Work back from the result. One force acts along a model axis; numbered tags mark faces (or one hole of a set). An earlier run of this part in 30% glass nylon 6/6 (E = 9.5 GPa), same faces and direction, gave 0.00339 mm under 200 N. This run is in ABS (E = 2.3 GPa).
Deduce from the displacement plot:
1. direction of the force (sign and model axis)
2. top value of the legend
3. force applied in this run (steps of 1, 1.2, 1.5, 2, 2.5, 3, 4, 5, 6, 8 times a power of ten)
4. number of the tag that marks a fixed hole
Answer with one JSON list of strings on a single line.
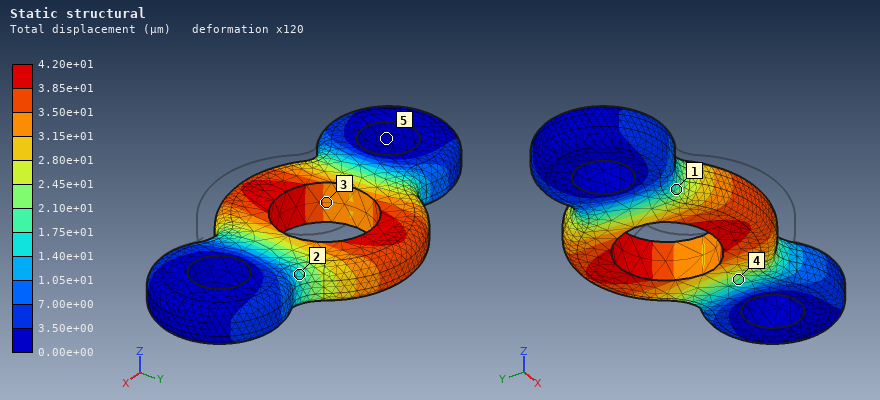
["+Y", "4.20e+01 µm", "600 N", "5"]
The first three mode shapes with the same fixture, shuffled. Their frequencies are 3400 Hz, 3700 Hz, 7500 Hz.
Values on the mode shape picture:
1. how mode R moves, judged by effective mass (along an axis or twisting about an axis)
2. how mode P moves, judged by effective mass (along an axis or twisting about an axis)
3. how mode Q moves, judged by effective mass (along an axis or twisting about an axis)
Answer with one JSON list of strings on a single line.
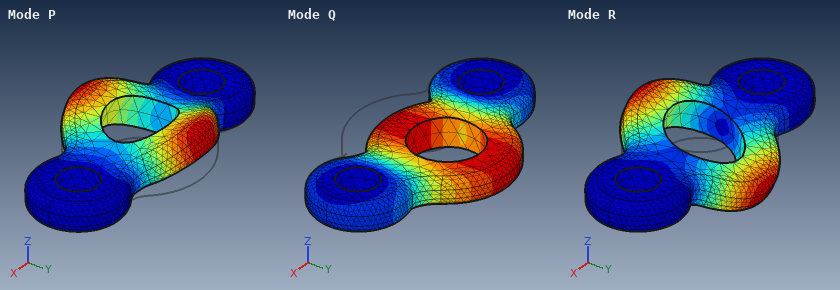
["twisting about X", "along Z", "along Y"]
